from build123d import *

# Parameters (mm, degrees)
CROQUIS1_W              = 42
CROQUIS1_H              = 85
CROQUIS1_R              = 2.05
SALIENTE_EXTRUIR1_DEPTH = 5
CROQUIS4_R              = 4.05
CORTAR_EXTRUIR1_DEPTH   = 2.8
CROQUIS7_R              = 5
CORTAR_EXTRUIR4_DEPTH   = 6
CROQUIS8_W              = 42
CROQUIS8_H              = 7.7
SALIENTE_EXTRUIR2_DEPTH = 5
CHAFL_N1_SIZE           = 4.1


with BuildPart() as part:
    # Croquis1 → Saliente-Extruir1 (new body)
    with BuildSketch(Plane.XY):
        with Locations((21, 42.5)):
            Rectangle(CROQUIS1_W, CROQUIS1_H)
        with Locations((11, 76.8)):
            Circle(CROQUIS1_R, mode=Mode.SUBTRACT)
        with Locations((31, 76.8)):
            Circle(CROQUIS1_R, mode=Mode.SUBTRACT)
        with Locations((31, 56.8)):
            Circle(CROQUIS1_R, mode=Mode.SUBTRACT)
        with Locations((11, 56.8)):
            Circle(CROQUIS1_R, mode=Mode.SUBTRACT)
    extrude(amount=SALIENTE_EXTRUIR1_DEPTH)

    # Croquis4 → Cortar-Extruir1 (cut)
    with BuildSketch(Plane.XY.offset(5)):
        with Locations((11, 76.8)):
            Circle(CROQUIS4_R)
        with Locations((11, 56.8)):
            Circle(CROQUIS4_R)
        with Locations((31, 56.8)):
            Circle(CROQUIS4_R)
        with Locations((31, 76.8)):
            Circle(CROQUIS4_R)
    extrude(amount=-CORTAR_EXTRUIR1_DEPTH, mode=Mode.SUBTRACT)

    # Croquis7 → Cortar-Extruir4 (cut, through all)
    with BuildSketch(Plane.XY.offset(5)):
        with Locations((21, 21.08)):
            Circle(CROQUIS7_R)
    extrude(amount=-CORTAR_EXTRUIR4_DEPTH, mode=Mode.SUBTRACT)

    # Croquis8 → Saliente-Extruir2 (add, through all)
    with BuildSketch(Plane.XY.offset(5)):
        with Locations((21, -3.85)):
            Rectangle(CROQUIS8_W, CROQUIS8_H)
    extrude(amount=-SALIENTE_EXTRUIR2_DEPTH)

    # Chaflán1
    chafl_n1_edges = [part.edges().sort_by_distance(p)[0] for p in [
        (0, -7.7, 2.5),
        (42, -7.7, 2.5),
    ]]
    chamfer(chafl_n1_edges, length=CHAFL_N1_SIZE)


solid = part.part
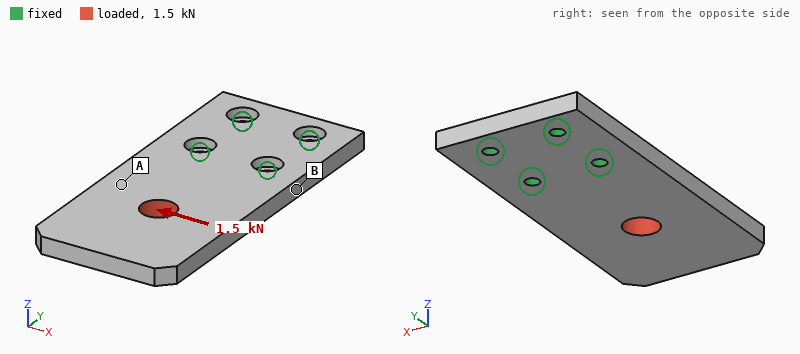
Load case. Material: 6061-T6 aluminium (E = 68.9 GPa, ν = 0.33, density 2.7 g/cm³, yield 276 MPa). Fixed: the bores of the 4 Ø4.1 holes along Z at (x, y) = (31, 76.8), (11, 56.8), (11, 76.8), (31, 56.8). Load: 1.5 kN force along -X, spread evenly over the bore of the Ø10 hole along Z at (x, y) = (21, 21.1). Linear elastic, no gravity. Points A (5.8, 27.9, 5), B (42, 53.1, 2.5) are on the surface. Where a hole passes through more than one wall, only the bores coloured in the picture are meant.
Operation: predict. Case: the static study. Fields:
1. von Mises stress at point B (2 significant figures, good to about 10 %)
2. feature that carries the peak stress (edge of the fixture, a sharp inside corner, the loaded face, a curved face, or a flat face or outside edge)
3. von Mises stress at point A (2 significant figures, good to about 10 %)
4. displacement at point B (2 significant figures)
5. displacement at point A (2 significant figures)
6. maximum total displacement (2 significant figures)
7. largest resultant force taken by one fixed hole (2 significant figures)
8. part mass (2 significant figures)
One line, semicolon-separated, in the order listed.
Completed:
31 MPa; edge of the fixture; 10 MPa; 11 µm; 29 µm; 60 µm; 1.7 kN; 49 g
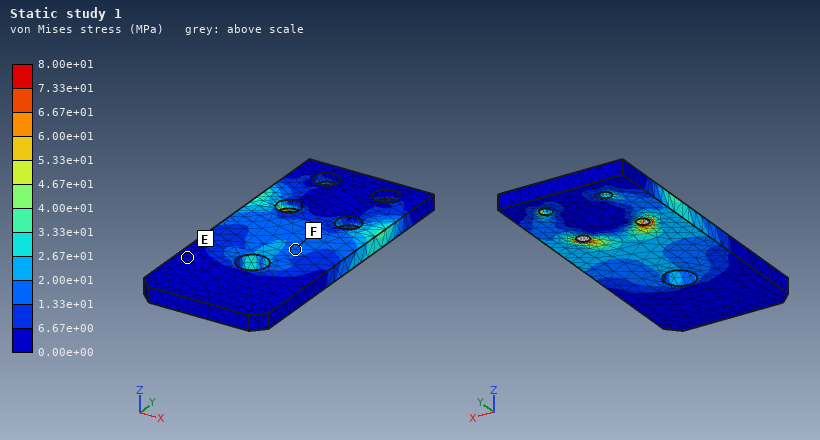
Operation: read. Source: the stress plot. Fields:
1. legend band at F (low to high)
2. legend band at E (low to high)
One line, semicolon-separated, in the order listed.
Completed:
1.33e+01 to 2.00e+01 MPa; 0.00e+00 to 6.67e+00 MPa
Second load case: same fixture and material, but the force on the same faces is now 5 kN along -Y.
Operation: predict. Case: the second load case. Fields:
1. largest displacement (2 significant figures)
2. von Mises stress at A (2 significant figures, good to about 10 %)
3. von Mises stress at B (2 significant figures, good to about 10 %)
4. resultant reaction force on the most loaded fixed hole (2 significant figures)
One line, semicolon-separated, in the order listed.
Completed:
90 µm; 17 MPa; 18 MPa; 1.8 kN
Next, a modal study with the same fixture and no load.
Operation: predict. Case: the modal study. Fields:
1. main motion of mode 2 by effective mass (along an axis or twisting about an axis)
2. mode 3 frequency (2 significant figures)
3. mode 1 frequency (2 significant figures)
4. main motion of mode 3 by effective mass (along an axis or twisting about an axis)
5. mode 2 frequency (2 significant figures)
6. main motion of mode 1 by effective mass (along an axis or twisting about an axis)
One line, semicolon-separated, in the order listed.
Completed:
twisting about Y; 5200 Hz; 880 Hz; along X; 3000 Hz; along Z
